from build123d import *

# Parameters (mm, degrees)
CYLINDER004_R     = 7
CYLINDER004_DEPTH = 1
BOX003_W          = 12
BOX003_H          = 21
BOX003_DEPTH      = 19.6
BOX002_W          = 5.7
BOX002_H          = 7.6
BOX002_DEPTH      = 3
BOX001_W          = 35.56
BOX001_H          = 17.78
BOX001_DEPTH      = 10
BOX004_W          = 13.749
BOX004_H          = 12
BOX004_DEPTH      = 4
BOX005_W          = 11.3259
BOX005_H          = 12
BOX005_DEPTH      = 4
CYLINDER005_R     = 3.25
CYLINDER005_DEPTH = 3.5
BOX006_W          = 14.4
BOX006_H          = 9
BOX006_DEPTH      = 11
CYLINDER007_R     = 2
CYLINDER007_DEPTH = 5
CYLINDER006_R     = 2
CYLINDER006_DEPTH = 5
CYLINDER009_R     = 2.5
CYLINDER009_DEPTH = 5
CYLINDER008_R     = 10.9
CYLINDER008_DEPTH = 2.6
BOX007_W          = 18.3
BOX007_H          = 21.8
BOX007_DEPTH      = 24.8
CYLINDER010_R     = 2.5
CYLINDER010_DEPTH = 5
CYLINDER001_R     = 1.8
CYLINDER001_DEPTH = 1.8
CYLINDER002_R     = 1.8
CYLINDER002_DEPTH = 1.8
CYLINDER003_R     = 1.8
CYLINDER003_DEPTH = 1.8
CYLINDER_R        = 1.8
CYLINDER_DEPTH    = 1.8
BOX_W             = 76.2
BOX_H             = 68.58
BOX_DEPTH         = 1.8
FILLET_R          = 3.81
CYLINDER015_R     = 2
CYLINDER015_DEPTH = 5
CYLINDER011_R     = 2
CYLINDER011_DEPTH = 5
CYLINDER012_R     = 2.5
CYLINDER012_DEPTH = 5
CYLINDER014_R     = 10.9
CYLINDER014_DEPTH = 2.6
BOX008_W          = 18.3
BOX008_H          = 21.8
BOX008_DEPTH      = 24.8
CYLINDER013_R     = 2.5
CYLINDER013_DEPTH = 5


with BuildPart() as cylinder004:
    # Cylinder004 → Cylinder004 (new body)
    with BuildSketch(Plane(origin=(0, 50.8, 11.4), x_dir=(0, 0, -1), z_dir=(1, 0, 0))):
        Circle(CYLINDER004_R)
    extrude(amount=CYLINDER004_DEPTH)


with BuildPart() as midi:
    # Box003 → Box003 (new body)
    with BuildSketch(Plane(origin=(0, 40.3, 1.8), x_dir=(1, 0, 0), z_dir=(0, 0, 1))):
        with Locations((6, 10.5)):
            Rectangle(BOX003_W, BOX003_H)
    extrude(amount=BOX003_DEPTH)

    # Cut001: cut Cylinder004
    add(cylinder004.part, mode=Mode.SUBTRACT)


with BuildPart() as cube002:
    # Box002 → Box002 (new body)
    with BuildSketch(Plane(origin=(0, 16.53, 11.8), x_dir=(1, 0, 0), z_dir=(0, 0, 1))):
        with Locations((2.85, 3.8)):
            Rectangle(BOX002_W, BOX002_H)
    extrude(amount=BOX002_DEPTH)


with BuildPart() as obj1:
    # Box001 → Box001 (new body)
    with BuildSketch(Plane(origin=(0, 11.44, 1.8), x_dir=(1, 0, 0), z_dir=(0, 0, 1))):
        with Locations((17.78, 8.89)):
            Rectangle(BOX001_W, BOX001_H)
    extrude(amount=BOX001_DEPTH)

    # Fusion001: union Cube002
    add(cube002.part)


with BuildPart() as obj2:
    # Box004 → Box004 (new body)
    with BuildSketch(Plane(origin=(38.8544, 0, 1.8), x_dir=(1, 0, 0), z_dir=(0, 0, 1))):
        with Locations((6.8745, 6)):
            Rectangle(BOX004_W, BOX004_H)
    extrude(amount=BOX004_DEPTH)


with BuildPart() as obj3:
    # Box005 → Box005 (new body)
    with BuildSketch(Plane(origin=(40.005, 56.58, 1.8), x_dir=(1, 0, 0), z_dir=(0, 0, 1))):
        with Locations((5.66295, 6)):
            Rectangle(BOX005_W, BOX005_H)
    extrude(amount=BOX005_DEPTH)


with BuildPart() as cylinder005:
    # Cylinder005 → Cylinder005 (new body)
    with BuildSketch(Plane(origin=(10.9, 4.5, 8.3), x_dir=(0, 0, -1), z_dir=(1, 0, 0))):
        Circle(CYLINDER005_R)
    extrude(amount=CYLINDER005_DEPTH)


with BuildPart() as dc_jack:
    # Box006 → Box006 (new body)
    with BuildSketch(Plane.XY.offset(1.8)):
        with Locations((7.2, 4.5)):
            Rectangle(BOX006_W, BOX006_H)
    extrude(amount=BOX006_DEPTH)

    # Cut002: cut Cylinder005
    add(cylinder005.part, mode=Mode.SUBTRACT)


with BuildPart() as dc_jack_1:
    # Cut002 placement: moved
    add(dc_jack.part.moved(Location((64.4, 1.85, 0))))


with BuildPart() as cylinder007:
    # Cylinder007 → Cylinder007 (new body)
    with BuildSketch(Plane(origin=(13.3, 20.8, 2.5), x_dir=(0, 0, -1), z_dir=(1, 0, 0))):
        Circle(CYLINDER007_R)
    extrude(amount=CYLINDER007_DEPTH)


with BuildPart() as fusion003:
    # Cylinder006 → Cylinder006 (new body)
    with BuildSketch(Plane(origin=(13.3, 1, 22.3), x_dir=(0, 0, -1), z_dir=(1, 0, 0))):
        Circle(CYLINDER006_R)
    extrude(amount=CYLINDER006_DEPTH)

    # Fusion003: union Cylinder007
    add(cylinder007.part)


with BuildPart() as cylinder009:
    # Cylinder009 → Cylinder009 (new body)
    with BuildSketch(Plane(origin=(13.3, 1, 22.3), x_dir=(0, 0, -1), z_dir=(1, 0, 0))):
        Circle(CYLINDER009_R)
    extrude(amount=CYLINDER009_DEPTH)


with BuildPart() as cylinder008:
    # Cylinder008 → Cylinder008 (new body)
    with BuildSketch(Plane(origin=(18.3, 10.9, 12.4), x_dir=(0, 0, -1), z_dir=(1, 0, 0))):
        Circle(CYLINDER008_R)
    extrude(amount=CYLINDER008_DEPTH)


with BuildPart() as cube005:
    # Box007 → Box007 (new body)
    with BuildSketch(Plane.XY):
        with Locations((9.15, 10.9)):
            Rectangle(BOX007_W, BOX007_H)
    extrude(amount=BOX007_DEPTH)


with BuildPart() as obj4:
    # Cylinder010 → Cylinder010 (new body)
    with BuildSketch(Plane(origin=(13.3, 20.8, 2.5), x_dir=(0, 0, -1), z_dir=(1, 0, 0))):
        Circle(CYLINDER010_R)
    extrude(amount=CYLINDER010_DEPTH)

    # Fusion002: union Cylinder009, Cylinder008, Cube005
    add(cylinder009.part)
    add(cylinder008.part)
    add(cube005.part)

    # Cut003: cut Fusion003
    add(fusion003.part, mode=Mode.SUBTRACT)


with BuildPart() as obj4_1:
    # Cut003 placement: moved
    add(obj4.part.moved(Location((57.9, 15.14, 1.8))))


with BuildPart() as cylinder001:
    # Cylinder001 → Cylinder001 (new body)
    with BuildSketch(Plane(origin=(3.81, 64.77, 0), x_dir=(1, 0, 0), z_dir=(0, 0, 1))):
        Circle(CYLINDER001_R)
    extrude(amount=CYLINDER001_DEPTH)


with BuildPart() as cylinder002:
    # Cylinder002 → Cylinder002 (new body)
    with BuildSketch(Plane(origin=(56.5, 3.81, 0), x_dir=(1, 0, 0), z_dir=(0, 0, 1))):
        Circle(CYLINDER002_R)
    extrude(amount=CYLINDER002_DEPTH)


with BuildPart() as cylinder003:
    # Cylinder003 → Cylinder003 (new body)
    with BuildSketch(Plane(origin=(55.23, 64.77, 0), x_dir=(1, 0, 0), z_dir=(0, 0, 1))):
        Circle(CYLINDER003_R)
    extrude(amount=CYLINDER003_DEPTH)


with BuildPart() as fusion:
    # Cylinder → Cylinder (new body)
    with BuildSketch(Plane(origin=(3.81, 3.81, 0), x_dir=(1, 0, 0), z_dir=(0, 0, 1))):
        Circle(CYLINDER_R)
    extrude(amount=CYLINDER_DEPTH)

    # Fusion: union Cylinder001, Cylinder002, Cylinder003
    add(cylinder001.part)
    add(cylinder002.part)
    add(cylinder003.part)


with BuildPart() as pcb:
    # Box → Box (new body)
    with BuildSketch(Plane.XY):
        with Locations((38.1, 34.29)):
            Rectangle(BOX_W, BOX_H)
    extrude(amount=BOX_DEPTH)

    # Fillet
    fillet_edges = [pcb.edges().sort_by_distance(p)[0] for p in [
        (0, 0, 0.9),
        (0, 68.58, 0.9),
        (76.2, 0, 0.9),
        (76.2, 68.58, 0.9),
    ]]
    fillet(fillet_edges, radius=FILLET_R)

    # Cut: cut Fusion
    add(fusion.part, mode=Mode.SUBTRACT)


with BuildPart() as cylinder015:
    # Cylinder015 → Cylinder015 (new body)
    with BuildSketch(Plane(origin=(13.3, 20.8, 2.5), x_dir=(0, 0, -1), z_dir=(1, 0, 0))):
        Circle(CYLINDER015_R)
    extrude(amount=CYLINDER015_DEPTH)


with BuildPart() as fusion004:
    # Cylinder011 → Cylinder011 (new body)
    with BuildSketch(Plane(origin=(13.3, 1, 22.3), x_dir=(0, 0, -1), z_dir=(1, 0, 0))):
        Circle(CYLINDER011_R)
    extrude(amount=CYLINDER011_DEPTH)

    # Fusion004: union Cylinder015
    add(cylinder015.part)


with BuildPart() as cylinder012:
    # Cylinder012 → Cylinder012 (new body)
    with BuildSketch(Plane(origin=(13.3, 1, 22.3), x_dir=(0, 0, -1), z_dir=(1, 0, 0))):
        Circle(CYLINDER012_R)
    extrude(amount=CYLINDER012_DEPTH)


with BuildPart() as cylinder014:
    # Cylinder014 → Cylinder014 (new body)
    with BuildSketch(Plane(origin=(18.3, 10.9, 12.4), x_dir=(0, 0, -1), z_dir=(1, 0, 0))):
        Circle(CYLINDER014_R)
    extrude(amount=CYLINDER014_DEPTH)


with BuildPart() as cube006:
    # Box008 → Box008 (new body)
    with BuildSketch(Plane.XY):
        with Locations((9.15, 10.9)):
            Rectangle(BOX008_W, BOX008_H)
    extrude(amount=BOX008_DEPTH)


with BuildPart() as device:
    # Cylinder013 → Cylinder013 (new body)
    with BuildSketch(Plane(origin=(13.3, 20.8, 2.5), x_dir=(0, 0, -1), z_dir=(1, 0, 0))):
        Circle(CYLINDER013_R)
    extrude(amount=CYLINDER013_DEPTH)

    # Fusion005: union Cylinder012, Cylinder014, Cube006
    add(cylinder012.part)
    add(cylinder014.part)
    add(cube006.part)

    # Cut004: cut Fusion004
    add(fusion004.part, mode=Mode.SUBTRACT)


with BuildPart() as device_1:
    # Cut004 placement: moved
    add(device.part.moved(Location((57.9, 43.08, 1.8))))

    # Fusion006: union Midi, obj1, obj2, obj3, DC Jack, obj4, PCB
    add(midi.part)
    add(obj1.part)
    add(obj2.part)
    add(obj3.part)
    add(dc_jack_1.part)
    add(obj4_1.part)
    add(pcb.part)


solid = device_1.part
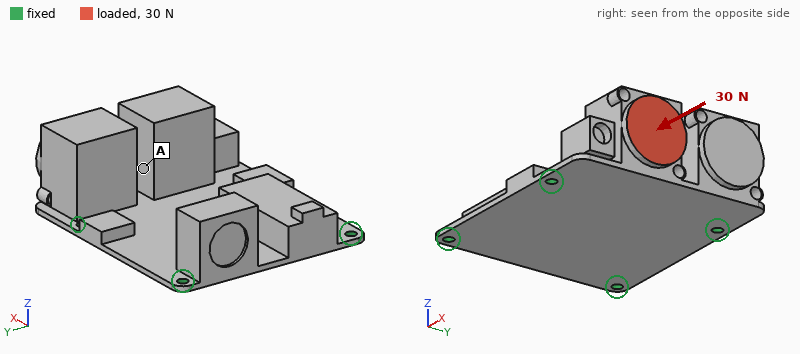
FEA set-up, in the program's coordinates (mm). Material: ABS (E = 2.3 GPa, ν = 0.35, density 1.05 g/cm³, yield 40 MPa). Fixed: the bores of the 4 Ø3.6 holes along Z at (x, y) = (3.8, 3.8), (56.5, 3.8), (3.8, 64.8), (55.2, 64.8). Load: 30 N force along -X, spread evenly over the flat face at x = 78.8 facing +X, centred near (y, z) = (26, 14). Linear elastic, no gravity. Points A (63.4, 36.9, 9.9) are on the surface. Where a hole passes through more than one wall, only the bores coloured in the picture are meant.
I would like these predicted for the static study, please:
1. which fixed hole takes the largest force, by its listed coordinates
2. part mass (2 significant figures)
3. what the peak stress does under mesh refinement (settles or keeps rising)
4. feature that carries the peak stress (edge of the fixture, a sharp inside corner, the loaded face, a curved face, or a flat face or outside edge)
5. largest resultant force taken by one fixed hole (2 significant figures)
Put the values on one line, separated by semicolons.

(56.5, 3.8); 47 g; keeps rising; edge of the fixture; 11 N
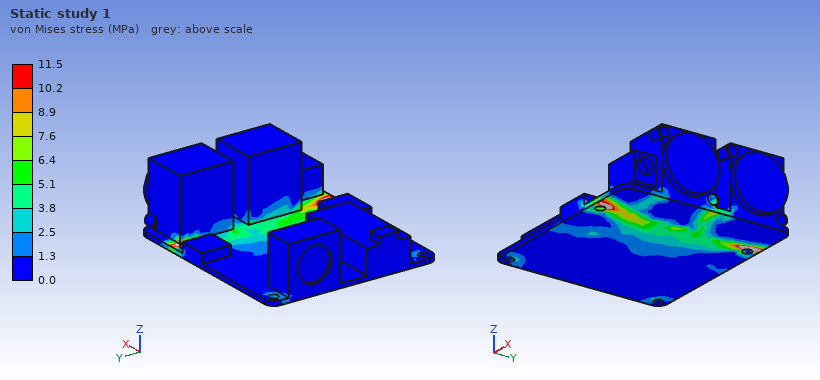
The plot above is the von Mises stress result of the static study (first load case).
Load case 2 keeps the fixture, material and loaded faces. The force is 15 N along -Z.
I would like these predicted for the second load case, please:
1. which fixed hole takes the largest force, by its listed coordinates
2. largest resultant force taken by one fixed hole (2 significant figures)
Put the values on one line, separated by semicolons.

(56.5, 3.8); 12 N
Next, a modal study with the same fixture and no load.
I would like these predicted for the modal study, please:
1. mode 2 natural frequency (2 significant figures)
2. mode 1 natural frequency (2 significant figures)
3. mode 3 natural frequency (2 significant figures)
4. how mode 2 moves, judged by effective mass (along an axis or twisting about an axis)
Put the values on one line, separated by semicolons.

330 Hz; 160 Hz; 490 Hz; along Z
